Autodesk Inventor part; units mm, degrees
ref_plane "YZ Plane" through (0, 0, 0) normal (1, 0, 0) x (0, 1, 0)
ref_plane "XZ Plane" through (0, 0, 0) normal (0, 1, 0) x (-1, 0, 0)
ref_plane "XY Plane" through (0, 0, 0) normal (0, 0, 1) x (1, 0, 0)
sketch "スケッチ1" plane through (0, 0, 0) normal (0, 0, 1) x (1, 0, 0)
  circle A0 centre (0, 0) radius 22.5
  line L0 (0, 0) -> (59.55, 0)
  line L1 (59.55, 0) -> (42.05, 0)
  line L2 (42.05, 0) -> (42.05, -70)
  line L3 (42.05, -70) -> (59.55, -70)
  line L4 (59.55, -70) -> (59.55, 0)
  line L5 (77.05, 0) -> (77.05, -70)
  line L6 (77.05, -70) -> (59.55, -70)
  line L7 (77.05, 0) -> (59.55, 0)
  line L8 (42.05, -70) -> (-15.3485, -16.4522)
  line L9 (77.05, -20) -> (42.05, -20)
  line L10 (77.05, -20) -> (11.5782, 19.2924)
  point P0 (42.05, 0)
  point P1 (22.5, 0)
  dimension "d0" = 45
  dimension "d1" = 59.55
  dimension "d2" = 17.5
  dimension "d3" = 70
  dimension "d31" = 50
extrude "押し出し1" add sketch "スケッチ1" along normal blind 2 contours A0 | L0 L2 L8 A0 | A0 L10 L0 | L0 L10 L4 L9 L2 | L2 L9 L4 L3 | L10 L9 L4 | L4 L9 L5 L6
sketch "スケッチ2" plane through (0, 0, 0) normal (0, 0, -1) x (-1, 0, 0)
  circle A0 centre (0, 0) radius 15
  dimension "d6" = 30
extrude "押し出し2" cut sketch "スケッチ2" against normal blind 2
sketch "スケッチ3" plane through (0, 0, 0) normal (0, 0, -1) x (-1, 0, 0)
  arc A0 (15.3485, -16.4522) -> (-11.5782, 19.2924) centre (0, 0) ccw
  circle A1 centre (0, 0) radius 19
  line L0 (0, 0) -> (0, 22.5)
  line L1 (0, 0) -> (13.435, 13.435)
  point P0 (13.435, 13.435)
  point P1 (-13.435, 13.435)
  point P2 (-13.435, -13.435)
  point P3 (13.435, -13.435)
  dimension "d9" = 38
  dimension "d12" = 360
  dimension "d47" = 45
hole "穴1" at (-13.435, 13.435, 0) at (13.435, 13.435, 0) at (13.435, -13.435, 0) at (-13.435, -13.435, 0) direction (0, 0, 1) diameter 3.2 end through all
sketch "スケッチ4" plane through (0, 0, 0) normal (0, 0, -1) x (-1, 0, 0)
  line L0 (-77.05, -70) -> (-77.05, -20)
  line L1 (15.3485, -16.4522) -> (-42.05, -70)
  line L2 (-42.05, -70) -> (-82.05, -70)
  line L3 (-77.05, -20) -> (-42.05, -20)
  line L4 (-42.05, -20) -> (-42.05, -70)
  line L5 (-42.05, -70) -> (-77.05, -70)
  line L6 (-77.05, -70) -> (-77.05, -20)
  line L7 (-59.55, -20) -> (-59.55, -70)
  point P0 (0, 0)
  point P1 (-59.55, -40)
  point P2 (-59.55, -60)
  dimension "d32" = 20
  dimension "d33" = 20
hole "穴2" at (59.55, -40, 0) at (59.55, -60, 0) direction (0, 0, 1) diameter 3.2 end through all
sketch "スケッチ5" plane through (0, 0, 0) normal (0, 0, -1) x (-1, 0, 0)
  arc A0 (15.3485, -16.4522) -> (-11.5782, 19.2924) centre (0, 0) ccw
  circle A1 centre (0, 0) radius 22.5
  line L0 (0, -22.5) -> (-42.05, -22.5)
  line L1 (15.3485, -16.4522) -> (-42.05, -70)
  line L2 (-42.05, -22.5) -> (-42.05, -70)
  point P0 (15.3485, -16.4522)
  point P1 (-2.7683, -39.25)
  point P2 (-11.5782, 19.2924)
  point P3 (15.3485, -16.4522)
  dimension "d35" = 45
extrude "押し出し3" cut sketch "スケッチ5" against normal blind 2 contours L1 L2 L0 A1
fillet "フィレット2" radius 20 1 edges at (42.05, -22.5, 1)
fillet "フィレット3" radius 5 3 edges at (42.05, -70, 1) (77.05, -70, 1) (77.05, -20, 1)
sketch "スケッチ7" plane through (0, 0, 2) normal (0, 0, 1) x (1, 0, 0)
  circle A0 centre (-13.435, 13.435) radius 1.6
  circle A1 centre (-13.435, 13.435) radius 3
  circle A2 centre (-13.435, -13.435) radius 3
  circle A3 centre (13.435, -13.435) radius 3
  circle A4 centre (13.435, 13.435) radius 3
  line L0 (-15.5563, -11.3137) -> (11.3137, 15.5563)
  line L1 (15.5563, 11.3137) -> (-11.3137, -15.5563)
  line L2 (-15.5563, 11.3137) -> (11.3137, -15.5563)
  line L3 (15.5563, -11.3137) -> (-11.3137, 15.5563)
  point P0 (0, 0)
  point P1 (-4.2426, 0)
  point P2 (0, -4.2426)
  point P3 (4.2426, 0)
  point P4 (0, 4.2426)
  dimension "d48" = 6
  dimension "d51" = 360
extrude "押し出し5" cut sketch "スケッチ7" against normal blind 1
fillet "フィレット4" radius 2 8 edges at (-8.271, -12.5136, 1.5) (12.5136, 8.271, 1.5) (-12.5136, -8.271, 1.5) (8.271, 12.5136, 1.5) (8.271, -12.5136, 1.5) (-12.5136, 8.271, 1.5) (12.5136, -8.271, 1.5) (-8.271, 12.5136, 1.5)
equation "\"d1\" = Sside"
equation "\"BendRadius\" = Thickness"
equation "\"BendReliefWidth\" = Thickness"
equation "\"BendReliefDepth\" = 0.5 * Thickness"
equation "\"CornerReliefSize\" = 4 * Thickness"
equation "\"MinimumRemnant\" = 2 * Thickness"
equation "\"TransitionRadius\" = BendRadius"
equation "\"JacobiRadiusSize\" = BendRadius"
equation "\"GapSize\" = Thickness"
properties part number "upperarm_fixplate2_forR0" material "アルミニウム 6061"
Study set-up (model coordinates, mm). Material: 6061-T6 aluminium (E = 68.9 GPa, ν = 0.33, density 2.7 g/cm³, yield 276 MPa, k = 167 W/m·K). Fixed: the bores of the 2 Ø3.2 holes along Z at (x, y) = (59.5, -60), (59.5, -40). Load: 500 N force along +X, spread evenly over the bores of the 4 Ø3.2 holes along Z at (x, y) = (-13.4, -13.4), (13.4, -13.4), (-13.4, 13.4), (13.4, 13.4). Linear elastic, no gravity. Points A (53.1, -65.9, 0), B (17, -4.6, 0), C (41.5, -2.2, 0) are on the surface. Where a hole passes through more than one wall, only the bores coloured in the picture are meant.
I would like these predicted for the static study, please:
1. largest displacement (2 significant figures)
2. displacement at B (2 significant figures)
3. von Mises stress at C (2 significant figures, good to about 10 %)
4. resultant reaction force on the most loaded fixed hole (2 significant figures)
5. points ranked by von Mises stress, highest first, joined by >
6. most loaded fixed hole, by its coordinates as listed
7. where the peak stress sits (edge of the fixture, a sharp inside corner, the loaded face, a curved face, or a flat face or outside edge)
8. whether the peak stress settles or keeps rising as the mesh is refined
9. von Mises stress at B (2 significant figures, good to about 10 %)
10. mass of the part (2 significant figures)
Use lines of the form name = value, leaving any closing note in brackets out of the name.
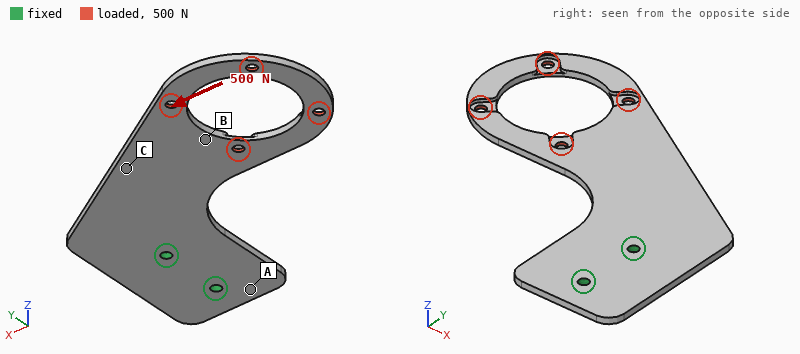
largest displacement = 0.78 mm
displacement at B = 0.25 mm
von Mises stress at C = 37 MPa
resultant reaction force on the most loaded fixed hole = 1.4 kN
points ranked by von Mises stress, highest first, joined by > = C > B > A
most loaded fixed hole, by its coordinates as listed = (59.5, -40)
where the peak stress sits = edge of the fixture
whether the peak stress settles or keeps rising as the mesh is refined = keeps rising
von Mises stress at B = 17 MPa
mass of the part = 20 g
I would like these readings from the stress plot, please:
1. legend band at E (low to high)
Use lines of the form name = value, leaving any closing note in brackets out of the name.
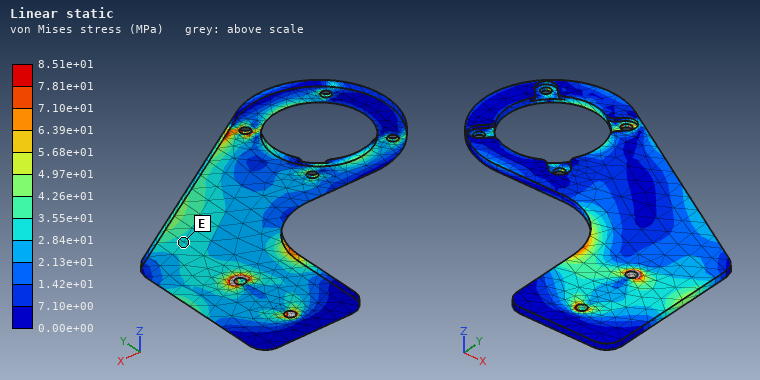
legend band at E = 2.84e+01 to 3.55e+01 MPa
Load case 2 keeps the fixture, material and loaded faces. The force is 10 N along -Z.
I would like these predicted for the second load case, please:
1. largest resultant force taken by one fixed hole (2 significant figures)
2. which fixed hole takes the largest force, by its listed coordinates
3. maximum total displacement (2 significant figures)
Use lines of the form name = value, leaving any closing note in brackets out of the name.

largest resultant force taken by one fixed hole = 19 N
which fixed hole takes the largest force, by its listed coordinates = (59.5, -40)
maximum total displacement = 1.4 mm
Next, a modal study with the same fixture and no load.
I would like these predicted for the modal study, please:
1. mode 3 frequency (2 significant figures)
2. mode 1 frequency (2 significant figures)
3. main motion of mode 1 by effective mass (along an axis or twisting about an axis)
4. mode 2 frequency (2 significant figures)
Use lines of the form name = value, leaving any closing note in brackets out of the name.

mode 3 frequency = 1000 Hz
mode 1 frequency = 220 Hz
main motion of mode 1 by effective mass = along Z
mode 2 frequency = 720 Hz
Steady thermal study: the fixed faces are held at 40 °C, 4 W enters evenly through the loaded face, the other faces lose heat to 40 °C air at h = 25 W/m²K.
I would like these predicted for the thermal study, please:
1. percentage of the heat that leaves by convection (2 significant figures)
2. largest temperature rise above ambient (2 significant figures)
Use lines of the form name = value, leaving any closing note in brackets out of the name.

percentage of the heat that leaves by convection = 46 %
largest temperature rise above ambient = 28 K
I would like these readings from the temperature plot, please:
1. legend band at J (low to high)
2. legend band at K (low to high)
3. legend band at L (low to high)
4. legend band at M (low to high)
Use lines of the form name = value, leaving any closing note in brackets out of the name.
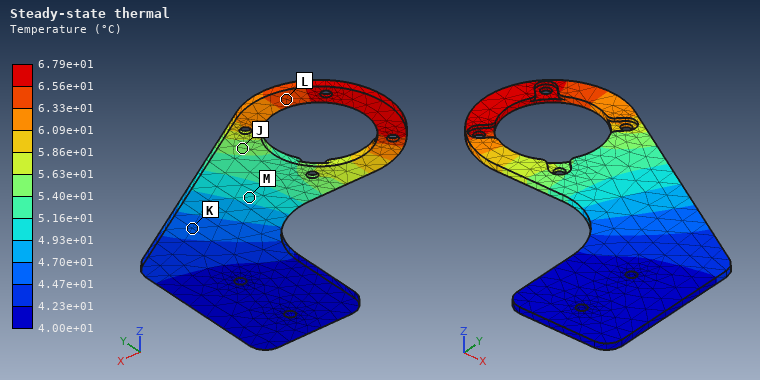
legend band at J = 5.40e+01 to 5.63e+01 °C
legend band at K = 4.47e+01 to 4.70e+01 °C
legend band at L = 6.33e+01 to 6.56e+01 °C
legend band at M = 4.93e+01 to 5.16e+01 °C
